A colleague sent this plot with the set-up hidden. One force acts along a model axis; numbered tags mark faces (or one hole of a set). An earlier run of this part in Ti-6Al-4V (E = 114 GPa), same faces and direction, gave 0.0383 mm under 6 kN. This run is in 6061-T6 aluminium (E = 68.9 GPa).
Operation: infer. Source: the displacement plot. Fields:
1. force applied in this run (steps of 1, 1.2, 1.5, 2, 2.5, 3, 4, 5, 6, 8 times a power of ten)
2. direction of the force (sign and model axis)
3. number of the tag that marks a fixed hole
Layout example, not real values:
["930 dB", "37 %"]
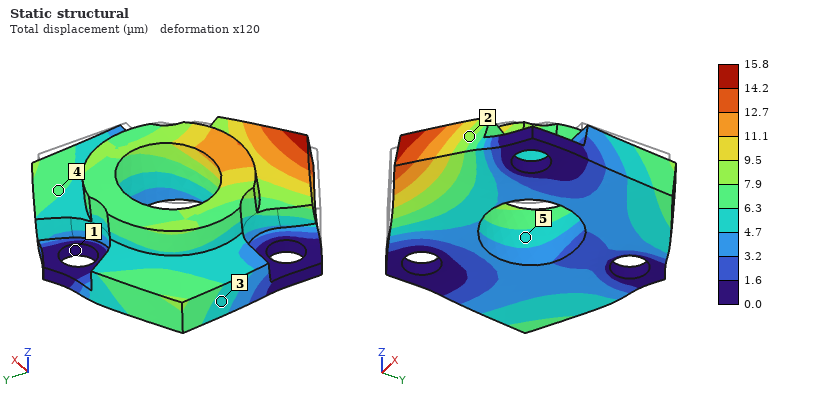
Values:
["1.5 kN", "+Y", "1"]
